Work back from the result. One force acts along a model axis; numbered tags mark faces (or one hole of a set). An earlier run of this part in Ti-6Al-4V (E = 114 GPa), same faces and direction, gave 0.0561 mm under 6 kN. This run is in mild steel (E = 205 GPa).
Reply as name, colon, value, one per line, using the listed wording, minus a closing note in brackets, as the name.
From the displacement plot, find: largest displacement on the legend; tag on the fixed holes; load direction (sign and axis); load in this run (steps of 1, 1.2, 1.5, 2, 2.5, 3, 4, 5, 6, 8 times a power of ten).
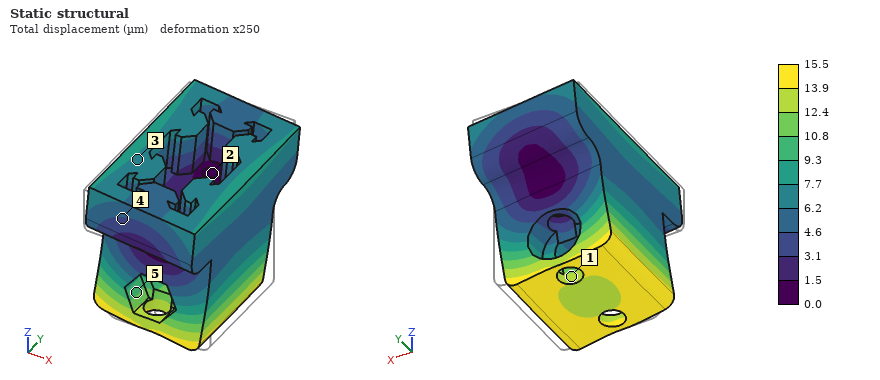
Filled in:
largest displacement on the legend: 15.5 µm
tag on the fixed holes: 2
load direction: -X
load in this run: 3 kN
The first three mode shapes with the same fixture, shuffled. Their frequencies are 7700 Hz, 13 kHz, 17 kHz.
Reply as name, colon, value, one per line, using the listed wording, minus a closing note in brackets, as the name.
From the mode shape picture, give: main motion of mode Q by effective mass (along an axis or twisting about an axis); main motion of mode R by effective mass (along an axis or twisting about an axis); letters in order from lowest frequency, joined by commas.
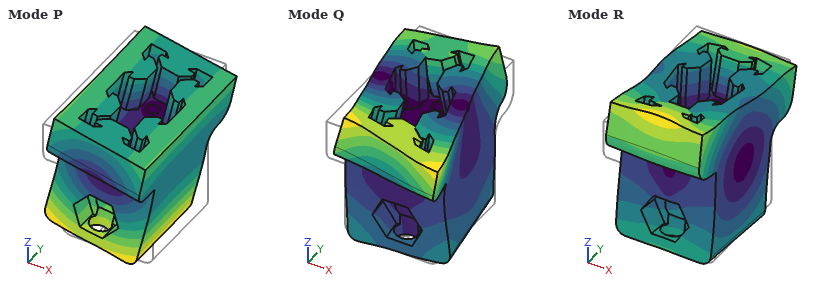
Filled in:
main motion of mode Q by effective mass: twisting about Z
main motion of mode R by effective mass: twisting about X
letters in order from lowest frequency, joined by commas: P, R, Q
